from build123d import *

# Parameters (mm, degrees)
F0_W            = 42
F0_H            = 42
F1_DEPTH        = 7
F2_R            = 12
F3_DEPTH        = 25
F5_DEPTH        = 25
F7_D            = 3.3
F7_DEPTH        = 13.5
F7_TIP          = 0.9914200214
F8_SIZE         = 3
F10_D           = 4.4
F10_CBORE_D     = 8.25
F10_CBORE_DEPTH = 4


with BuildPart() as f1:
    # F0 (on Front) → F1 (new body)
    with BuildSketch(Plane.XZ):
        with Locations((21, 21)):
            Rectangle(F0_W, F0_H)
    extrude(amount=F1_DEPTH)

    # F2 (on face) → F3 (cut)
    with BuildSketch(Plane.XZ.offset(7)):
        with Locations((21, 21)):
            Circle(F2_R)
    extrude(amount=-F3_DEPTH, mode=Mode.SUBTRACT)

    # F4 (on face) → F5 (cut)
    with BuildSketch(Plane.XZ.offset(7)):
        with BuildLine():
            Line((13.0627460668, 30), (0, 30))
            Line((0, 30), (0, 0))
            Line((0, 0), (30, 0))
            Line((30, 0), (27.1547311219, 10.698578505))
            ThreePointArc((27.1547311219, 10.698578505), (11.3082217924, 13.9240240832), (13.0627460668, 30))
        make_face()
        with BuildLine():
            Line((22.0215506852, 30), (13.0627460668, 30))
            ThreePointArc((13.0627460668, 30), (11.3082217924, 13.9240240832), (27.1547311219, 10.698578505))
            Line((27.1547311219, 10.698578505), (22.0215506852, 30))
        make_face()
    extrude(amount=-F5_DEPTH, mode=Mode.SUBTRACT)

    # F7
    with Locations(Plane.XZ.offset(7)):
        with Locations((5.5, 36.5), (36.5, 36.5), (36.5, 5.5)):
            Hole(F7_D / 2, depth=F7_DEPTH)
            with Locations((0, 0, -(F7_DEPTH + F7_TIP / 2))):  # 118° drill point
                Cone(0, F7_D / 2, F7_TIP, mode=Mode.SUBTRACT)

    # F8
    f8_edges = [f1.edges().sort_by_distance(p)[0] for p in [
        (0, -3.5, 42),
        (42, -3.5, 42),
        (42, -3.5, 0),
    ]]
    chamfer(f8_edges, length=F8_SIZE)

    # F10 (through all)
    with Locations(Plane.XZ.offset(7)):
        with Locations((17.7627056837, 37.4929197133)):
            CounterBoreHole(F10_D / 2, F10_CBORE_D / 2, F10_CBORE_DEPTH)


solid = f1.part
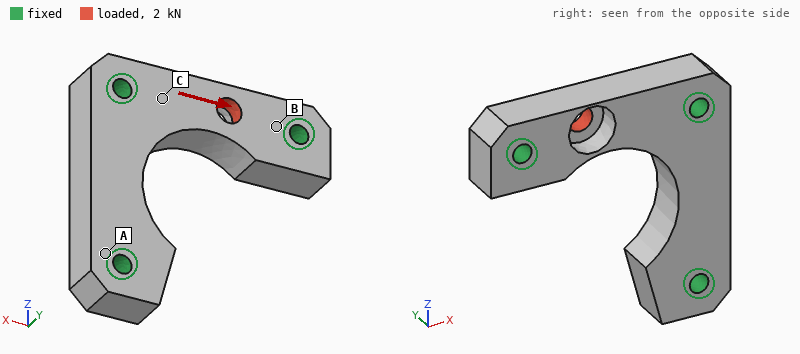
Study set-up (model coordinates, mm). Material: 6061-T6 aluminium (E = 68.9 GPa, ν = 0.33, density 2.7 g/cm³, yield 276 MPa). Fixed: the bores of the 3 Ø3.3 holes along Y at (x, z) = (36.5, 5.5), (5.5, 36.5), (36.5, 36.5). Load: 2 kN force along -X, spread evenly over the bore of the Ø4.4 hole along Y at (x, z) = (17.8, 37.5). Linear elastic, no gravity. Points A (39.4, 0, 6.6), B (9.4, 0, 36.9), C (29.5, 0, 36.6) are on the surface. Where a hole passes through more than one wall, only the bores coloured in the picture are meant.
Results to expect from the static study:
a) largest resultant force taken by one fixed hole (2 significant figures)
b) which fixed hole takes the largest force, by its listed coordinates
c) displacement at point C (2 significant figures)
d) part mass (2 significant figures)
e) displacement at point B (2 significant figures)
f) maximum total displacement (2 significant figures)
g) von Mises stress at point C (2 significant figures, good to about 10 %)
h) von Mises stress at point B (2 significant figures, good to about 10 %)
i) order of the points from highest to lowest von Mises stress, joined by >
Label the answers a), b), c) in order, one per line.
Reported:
a) 1.1 kN
b) (5.5, 36.5)
c) 1.3 µm
d) 14 g
e) 1.3 µm
f) 6.0 µm
g) 18 MPa
h) 38 MPa
i) B > C > A
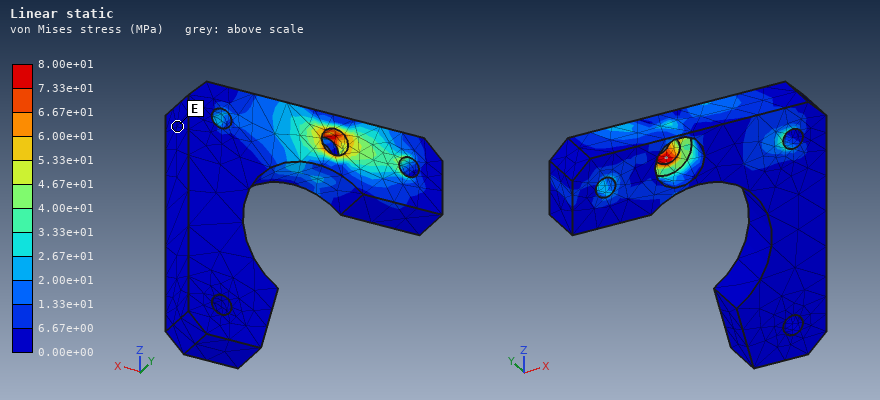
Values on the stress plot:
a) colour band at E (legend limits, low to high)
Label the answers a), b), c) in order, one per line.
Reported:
a) 0.00e+00 to 6.67e+00 MPa
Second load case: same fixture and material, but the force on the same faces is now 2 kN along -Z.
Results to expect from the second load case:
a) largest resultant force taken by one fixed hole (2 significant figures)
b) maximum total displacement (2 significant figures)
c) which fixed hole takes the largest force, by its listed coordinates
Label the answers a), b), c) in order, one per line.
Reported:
a) 1.1 kN
b) 28 µm
c) (5.5, 36.5)
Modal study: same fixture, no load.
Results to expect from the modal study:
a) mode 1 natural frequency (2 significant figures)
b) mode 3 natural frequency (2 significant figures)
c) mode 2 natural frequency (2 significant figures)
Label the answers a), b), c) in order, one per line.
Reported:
a) 28 kHz
b) 31 kHz
c) 30 kHz
